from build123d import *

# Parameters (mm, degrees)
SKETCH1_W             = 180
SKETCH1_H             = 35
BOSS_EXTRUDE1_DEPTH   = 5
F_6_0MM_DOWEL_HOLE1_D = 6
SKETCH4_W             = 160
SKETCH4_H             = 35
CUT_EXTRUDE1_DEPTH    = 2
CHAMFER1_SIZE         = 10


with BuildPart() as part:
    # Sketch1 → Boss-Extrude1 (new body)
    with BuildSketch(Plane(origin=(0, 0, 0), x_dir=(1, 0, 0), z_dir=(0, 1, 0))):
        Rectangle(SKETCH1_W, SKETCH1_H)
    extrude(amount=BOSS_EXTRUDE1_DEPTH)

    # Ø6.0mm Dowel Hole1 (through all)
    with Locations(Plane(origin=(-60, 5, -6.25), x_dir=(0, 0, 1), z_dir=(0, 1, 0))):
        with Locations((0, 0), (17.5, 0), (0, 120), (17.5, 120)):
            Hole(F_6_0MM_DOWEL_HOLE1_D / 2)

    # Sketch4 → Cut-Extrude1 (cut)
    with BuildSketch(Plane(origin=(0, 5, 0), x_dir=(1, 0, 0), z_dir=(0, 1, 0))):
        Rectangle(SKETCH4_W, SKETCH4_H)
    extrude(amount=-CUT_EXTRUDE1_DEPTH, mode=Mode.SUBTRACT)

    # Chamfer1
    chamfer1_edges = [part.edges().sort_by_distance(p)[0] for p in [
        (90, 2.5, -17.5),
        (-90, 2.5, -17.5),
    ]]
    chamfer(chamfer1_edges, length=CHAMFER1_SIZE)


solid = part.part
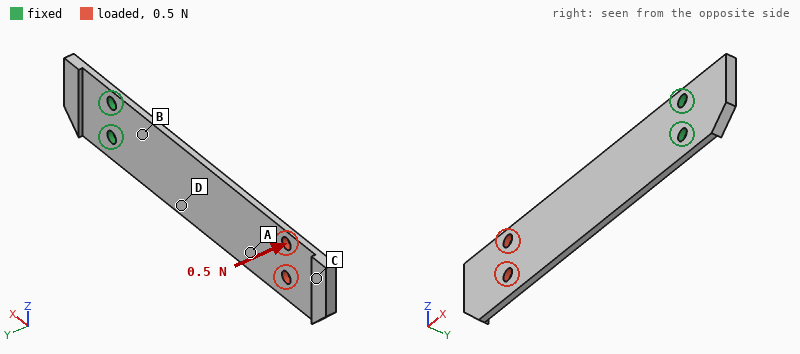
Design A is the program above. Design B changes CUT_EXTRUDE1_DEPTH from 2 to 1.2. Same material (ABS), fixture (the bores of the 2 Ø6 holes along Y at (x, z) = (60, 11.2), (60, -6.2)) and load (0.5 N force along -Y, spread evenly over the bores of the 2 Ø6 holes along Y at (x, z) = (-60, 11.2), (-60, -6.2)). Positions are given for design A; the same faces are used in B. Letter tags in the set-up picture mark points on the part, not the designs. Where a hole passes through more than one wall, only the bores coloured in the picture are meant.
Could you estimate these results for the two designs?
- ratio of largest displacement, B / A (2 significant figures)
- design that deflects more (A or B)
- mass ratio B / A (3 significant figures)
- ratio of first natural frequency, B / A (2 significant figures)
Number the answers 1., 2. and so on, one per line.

1. 0.49
2. A
3. 1.23
4. 1.3
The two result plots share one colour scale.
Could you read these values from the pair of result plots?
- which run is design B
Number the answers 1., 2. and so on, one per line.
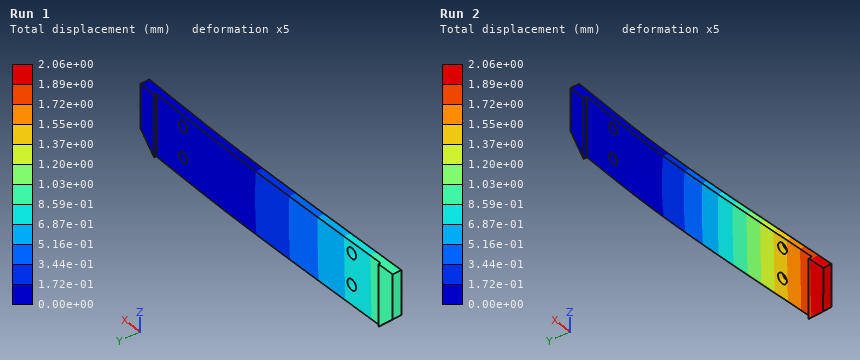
1. Run 1
